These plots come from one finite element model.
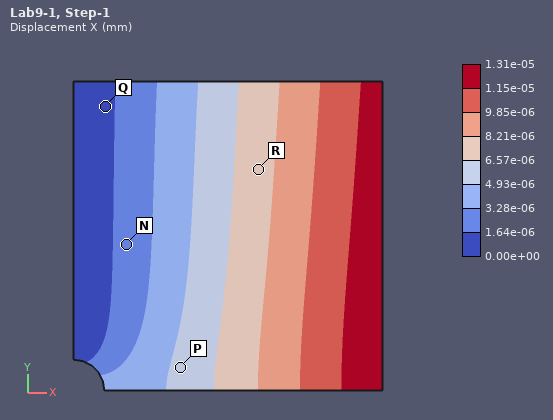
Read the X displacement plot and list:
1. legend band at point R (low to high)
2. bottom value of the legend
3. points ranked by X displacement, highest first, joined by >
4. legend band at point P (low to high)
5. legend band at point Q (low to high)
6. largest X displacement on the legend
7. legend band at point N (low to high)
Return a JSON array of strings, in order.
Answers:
["6.57e-06 to 8.21e-06 mm", "0.00e+00 mm", "R > P > N > Q", "4.93e-06 to 6.57e-06 mm", "0.00e+00 to 1.64e-06 mm", "1.31e-05 mm", "1.64e-06 to 3.28e-06 mm"]
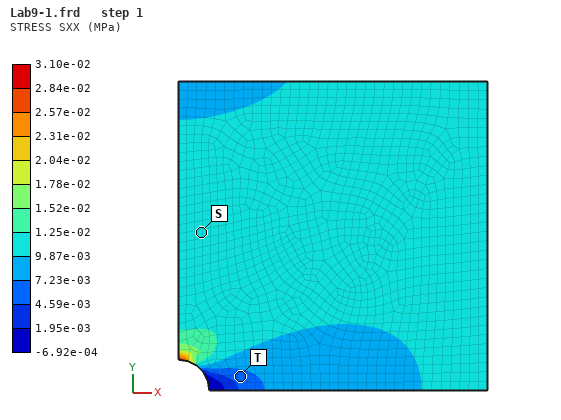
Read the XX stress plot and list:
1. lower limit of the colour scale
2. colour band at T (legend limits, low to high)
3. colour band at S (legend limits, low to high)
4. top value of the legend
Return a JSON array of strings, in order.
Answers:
["-6.92e-04 MPa", "4.59e-03 to 7.23e-03 MPa", "9.87e-03 to 1.25e-02 MPa", "3.10e-02 MPa"]
